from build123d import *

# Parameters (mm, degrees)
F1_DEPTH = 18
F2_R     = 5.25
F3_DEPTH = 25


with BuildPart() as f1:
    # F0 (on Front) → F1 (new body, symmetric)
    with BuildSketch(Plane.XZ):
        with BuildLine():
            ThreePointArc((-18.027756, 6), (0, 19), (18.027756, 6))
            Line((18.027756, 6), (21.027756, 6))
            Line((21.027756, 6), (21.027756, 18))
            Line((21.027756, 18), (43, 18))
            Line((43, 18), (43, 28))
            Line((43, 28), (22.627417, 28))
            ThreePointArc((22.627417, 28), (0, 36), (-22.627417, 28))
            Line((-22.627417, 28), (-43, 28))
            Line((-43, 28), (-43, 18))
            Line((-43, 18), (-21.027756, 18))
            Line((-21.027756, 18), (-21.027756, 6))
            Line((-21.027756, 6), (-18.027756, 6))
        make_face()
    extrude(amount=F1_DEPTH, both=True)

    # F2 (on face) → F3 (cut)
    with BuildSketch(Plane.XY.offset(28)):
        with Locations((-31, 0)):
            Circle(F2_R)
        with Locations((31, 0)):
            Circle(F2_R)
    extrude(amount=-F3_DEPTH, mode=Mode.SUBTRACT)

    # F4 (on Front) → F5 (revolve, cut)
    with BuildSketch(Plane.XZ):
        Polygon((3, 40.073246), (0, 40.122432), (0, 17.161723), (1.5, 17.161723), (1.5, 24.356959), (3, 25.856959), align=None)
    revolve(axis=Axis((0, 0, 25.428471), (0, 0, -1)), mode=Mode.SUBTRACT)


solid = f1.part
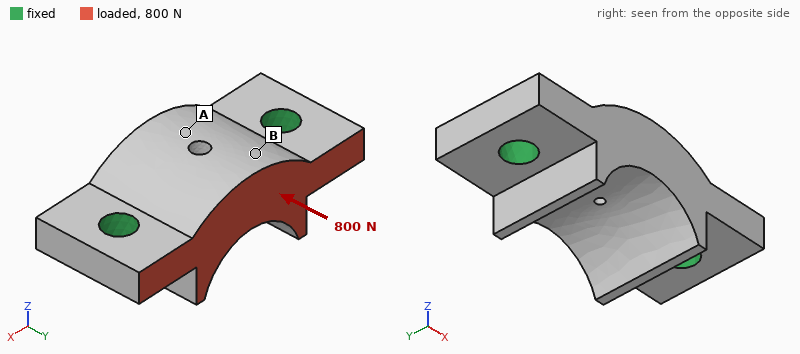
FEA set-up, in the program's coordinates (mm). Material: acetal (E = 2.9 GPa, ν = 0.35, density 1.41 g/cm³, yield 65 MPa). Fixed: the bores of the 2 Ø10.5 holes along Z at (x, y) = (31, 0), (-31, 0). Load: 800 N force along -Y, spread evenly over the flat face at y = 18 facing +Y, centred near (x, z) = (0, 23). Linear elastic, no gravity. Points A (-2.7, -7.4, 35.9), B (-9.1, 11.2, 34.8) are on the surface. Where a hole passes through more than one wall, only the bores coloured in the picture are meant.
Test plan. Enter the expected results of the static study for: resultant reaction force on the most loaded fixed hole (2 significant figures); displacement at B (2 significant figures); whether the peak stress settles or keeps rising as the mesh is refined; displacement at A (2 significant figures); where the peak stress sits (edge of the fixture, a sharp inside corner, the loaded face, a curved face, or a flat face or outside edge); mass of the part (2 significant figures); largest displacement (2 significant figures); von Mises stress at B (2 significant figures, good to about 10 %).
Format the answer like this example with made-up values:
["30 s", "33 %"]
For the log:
["400 N", "21 µm", "keeps rising", "20 µm", "edge of the fixture", "61 g", "26 µm", "0.69 MPa"]
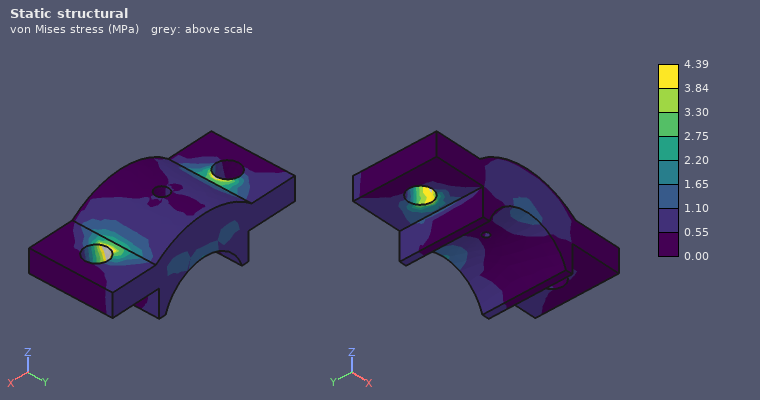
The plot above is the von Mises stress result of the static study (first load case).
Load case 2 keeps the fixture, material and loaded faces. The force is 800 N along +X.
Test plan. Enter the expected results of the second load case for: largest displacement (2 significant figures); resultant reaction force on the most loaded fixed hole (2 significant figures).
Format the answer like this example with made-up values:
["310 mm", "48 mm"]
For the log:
["33 µm", "450 N"]
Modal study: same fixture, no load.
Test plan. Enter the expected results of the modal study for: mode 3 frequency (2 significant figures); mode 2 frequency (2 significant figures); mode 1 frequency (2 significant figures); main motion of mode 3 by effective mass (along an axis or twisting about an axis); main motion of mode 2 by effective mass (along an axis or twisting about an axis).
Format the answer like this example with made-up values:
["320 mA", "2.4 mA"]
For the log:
["4600 Hz", "3500 Hz", "3100 Hz", "along Y", "along Z"]
